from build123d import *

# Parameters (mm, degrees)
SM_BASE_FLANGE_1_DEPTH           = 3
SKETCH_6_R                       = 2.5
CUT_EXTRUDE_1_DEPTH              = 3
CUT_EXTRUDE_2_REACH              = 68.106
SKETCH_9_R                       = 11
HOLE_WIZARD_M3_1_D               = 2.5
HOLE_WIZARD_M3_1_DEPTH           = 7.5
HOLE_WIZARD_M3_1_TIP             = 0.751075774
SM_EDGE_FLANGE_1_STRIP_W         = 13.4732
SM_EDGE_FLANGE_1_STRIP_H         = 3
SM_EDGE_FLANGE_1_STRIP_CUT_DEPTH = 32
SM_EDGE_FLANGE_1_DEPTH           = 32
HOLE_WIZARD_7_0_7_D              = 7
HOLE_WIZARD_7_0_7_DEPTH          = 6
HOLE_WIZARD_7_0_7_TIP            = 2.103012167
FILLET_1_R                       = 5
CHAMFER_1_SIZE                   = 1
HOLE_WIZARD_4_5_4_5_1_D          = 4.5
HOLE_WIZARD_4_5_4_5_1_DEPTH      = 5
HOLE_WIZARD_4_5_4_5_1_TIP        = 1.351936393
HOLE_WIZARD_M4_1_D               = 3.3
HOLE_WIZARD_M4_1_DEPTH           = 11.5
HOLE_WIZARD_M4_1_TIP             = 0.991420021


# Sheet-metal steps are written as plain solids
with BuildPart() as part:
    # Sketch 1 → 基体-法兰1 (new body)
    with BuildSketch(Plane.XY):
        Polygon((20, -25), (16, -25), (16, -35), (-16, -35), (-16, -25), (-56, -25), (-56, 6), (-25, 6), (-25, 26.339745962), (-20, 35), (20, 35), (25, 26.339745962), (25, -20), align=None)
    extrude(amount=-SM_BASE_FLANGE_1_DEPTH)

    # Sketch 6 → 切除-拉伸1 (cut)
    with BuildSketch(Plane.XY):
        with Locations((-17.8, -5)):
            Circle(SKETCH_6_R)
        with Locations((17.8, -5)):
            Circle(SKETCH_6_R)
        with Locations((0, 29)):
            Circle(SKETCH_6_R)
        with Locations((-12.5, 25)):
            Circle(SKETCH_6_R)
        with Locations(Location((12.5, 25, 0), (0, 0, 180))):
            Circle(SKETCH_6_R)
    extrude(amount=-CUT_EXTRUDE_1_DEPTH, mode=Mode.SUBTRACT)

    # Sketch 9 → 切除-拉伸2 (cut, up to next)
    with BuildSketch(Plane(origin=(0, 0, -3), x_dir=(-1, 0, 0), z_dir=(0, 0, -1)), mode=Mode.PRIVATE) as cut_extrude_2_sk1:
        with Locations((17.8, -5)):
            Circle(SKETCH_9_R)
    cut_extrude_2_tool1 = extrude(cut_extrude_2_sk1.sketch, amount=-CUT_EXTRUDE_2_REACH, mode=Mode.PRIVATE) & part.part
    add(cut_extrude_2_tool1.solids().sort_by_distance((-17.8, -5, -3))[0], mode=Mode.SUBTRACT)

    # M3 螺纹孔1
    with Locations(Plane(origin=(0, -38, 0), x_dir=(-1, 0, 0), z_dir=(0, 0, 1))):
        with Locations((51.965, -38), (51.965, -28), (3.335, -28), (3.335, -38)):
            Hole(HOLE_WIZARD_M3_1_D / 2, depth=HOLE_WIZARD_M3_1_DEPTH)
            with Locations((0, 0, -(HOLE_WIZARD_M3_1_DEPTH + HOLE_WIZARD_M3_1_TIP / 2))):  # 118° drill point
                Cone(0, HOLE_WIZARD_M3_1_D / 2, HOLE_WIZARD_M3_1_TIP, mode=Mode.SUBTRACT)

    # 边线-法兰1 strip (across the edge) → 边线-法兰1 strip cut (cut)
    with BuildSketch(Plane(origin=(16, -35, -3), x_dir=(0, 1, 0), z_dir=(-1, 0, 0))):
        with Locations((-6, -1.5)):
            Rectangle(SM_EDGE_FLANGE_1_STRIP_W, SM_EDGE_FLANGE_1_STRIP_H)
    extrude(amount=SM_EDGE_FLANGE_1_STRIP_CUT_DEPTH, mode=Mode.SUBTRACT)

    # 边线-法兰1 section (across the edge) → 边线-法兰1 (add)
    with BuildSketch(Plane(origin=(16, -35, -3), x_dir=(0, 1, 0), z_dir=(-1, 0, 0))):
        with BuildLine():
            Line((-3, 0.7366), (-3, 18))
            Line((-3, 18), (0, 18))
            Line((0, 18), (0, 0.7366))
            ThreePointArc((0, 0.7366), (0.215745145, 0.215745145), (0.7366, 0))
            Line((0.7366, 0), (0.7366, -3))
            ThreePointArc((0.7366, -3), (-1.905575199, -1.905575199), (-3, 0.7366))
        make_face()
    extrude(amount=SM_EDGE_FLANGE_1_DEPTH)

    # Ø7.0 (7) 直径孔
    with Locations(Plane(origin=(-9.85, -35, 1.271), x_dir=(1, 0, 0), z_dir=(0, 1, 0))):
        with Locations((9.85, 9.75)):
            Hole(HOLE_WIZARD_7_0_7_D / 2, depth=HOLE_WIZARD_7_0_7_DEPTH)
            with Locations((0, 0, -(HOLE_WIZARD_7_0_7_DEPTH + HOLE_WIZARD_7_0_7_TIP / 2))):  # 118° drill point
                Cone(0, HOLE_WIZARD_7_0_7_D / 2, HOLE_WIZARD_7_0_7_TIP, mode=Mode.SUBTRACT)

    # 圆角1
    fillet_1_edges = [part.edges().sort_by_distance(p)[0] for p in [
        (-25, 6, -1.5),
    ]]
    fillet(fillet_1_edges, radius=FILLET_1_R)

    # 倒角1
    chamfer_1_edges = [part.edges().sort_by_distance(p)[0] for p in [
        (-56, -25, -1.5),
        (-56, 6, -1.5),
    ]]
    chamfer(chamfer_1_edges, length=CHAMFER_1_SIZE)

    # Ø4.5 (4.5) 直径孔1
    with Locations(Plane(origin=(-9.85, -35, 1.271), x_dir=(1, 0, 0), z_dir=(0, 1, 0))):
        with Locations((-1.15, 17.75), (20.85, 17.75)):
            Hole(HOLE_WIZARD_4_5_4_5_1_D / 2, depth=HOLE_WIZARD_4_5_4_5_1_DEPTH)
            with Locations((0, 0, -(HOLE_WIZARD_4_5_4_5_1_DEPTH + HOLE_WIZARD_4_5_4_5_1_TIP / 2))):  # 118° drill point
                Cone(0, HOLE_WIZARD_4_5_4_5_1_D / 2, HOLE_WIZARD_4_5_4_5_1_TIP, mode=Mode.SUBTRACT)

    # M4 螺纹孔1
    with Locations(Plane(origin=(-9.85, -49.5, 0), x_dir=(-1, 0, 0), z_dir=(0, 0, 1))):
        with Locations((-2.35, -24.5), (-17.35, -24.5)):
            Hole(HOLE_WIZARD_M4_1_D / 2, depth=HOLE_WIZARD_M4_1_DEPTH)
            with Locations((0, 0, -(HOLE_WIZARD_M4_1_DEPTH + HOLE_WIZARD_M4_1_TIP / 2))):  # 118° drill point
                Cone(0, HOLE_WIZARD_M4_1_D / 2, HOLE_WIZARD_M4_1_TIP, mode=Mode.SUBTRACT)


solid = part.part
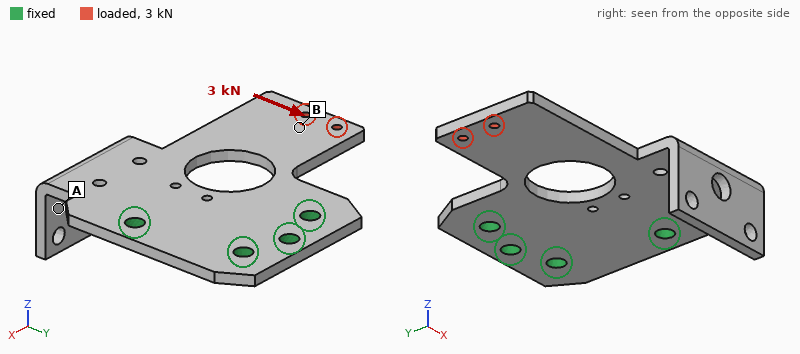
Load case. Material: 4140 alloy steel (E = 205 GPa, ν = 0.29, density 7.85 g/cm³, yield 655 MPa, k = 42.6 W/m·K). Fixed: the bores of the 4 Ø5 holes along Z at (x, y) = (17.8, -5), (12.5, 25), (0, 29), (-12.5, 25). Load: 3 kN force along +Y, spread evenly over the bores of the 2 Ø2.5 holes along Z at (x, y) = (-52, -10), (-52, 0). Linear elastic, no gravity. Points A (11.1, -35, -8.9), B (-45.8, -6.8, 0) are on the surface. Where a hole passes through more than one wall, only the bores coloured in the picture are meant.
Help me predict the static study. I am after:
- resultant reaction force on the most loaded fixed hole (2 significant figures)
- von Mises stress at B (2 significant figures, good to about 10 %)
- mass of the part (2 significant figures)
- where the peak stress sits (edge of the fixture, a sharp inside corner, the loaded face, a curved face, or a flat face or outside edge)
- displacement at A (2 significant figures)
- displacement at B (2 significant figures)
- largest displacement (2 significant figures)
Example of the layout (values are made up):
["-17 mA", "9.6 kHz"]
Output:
["3.4 kN", "82 MPa", "100 g", "a curved face", "0.028 mm", "0.072 mm", "0.10 mm"]
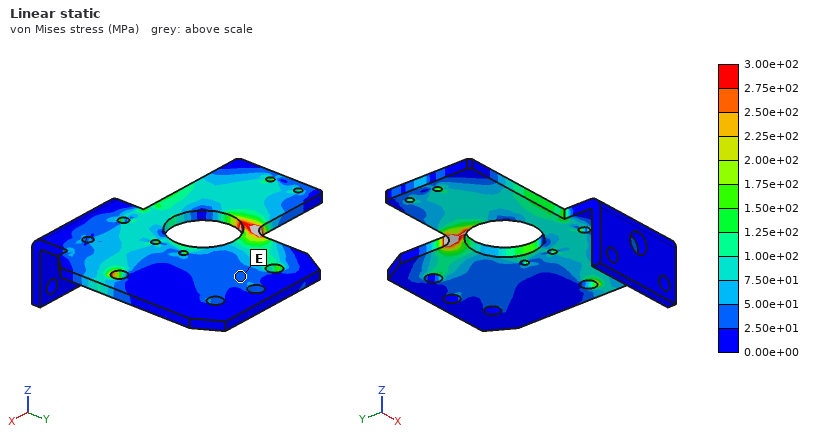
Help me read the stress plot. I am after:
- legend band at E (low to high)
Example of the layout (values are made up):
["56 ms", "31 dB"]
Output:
["2.50e+01 to 5.00e+01 MPa"]
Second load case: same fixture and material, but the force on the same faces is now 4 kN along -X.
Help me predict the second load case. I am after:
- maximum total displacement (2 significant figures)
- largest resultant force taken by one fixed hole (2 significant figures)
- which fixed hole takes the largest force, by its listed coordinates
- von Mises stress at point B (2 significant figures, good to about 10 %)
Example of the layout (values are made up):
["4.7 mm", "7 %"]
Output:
["37 µm", "2.9 kN", "(17.8, -5)", "54 MPa"]
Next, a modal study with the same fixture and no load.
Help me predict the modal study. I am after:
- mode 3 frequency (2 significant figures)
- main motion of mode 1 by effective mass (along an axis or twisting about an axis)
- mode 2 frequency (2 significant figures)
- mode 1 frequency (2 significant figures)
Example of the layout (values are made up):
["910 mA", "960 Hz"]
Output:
["2400 Hz", "along Z", "1200 Hz", "660 Hz"]
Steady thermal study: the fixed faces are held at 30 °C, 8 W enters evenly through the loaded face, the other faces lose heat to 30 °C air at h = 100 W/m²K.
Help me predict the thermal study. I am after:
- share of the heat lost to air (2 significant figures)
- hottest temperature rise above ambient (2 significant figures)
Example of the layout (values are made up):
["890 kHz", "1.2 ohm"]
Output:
["91 %", "54 K"]
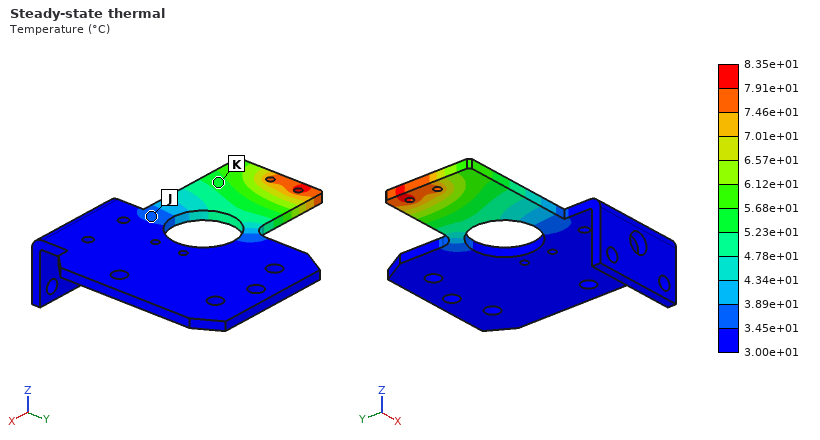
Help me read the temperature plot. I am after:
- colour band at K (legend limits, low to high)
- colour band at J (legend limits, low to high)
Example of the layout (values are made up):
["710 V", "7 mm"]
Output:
["5.23e+01 to 5.68e+01 °C", "3.45e+01 to 3.89e+01 °C"]
